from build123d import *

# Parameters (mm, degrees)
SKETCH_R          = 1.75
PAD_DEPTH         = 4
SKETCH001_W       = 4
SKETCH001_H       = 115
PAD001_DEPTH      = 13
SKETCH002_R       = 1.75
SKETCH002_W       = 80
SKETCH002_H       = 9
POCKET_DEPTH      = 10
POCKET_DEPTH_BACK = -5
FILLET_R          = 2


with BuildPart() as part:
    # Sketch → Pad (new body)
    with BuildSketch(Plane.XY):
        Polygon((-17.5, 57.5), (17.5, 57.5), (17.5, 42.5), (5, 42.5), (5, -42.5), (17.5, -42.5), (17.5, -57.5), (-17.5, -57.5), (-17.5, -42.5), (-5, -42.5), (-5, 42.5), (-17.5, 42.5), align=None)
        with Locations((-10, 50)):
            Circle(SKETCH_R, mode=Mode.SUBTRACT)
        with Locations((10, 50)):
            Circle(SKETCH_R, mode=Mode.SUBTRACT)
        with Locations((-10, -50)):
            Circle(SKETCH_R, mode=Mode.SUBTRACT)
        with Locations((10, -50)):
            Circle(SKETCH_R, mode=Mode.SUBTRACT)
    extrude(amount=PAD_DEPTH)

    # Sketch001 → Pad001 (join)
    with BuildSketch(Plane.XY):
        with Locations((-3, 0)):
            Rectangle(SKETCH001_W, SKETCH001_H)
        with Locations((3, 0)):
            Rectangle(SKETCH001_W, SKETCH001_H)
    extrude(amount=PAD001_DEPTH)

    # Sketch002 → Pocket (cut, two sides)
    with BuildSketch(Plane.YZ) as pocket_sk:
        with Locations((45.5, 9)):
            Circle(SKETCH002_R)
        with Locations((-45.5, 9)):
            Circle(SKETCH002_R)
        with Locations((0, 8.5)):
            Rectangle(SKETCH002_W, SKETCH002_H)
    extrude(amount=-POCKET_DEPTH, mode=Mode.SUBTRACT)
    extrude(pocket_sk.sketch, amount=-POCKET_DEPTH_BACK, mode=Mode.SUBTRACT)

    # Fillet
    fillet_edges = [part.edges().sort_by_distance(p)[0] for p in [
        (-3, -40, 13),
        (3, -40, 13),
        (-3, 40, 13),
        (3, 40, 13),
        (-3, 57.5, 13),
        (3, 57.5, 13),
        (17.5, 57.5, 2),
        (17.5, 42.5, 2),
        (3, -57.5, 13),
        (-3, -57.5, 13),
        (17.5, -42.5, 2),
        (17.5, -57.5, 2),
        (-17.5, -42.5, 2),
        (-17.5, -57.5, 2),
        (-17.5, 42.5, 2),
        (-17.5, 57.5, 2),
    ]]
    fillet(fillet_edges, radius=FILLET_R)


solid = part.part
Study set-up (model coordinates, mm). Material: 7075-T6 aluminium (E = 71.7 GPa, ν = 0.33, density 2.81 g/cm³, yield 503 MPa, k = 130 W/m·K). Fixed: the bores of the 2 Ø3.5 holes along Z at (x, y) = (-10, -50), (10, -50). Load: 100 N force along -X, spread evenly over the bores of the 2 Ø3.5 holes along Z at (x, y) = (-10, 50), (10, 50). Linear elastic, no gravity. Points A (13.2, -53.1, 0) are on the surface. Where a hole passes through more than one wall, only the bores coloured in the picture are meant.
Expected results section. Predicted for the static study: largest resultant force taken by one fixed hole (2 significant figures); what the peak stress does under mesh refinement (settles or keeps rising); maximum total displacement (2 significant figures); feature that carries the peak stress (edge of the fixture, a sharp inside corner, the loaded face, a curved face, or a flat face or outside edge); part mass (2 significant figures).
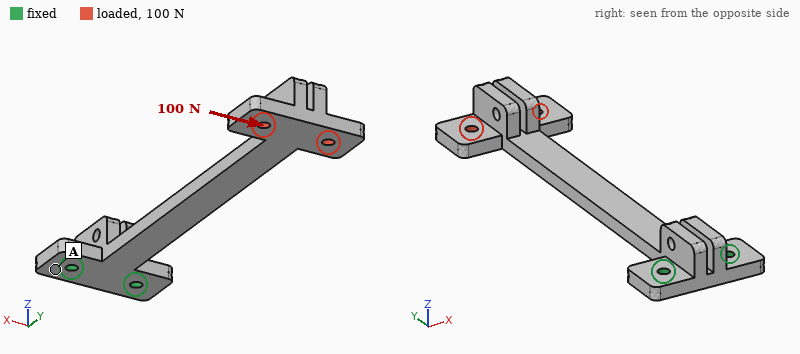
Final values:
520 N
keeps rising
1.4 mm
a sharp inside corner
27 g
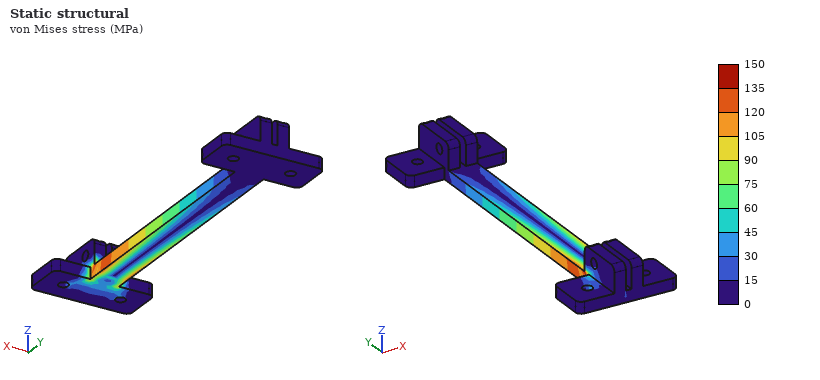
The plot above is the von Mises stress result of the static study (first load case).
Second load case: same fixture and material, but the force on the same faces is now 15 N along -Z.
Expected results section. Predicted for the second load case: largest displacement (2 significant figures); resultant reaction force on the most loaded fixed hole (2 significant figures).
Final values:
1.2 mm
30 N
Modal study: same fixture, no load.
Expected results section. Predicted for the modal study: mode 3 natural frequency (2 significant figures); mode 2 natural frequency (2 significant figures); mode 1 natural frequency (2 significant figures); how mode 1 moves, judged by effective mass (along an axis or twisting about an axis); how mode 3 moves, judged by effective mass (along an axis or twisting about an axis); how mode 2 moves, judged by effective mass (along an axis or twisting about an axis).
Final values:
1300 Hz
440 Hz
180 Hz
along Z
twisting about Y
along X
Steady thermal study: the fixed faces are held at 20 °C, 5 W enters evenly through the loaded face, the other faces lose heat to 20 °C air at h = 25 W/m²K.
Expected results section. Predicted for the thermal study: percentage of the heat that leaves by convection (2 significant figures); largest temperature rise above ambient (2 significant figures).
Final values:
64 %
41 K
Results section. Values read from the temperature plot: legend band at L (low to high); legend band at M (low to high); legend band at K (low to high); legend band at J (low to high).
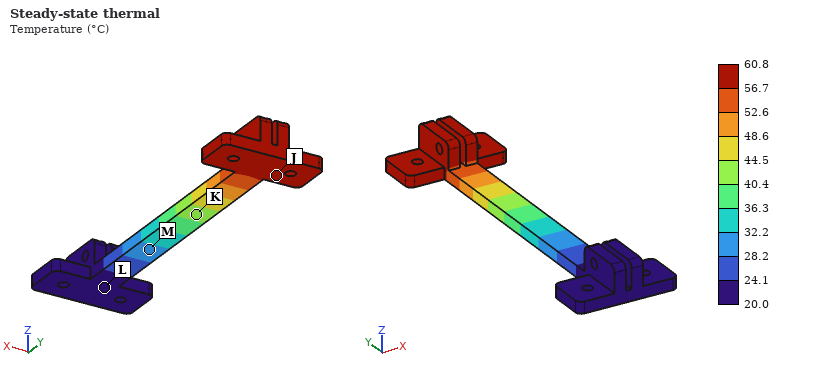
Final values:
20.0 to 24.1 °C
28.2 to 32.2 °C
40.4 to 44.5 °C
56.7 to 60.8 °C
